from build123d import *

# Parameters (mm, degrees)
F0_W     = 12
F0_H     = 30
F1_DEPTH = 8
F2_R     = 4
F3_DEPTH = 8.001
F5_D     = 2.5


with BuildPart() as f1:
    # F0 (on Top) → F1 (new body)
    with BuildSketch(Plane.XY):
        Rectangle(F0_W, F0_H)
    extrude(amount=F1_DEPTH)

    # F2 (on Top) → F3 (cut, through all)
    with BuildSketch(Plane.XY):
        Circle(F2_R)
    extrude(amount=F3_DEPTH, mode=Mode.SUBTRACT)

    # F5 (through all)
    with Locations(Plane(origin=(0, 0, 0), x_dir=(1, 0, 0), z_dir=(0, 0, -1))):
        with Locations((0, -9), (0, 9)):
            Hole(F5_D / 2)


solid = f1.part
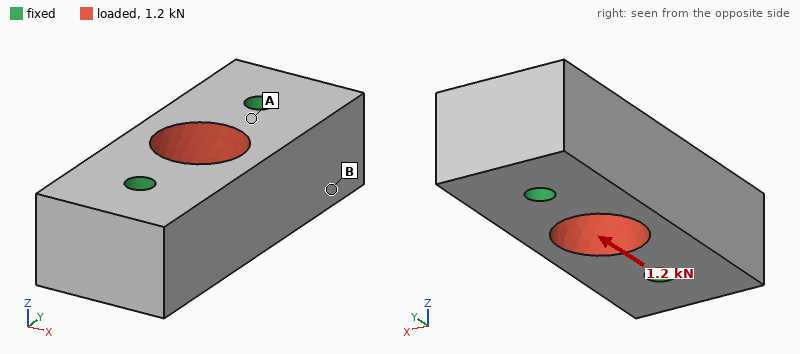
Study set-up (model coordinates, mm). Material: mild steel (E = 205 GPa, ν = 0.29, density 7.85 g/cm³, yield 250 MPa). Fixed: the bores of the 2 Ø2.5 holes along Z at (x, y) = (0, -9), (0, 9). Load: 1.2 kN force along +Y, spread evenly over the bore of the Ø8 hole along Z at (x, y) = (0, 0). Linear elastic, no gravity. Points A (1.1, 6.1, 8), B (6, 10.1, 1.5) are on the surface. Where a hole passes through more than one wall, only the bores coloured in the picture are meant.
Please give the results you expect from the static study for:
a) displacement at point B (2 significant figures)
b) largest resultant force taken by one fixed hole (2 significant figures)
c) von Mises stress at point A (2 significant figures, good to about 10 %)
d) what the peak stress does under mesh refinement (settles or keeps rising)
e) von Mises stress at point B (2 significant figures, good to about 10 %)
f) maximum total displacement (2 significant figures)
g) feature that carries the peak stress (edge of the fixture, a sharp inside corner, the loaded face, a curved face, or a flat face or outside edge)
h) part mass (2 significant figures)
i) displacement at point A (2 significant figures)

0.18 µm
600 N
9.8 MPa
keeps rising
3.0 MPa
0.42 µm
edge of the fixture
19 g
0.12 µm
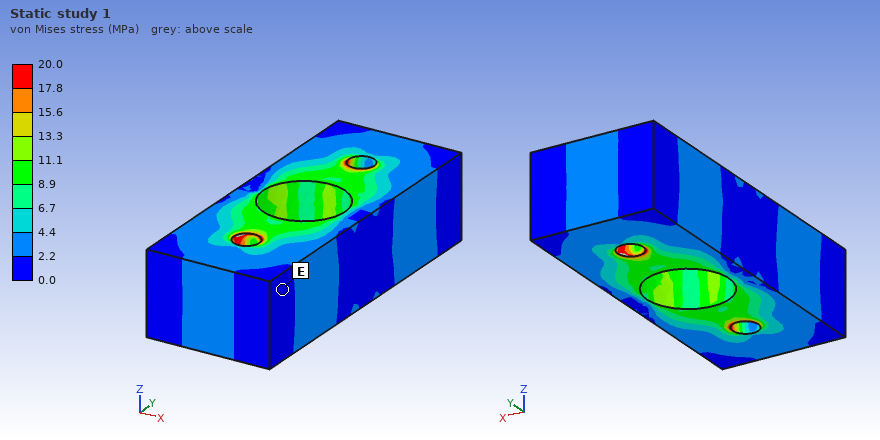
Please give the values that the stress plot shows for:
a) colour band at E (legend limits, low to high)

0.0 to 2.2 MPa
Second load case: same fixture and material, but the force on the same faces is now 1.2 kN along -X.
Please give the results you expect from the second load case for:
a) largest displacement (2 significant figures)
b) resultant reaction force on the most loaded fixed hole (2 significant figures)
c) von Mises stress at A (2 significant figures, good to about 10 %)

1.3 µm
600 N
18 MPa
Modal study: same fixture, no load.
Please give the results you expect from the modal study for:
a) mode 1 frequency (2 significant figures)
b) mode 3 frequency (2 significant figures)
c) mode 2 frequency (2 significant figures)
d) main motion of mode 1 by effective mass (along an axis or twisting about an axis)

53 kHz
66 kHz
64 kHz
twisting about Z
